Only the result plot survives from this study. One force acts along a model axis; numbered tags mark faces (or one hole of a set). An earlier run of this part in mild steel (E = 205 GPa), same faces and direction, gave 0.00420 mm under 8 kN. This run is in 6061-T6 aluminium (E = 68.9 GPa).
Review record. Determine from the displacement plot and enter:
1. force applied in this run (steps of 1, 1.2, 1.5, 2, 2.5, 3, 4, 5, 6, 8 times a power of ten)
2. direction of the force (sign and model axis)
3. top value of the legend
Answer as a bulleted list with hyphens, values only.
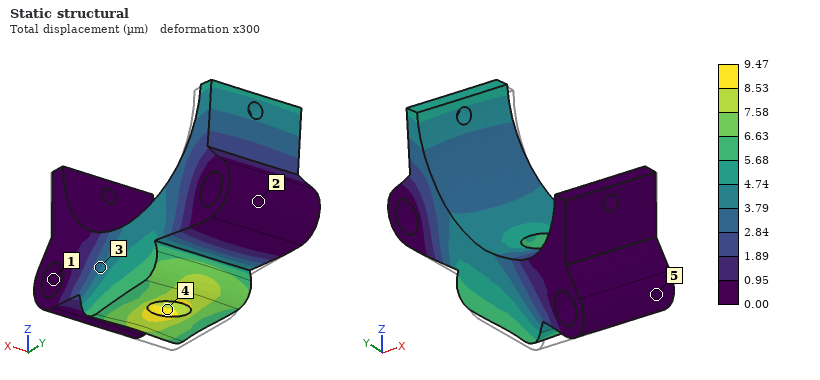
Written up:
- 6 kN
- +Y
- 9.47 µm
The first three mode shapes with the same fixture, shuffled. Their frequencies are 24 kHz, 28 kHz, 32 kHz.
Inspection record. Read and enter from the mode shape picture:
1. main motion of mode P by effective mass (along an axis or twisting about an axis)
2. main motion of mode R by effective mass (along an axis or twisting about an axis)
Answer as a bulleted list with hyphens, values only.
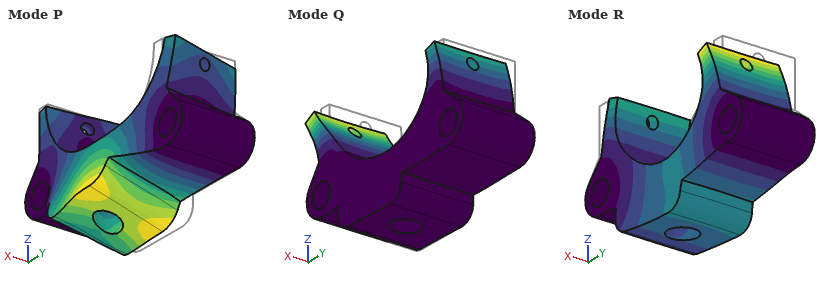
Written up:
- along X
- along Z
